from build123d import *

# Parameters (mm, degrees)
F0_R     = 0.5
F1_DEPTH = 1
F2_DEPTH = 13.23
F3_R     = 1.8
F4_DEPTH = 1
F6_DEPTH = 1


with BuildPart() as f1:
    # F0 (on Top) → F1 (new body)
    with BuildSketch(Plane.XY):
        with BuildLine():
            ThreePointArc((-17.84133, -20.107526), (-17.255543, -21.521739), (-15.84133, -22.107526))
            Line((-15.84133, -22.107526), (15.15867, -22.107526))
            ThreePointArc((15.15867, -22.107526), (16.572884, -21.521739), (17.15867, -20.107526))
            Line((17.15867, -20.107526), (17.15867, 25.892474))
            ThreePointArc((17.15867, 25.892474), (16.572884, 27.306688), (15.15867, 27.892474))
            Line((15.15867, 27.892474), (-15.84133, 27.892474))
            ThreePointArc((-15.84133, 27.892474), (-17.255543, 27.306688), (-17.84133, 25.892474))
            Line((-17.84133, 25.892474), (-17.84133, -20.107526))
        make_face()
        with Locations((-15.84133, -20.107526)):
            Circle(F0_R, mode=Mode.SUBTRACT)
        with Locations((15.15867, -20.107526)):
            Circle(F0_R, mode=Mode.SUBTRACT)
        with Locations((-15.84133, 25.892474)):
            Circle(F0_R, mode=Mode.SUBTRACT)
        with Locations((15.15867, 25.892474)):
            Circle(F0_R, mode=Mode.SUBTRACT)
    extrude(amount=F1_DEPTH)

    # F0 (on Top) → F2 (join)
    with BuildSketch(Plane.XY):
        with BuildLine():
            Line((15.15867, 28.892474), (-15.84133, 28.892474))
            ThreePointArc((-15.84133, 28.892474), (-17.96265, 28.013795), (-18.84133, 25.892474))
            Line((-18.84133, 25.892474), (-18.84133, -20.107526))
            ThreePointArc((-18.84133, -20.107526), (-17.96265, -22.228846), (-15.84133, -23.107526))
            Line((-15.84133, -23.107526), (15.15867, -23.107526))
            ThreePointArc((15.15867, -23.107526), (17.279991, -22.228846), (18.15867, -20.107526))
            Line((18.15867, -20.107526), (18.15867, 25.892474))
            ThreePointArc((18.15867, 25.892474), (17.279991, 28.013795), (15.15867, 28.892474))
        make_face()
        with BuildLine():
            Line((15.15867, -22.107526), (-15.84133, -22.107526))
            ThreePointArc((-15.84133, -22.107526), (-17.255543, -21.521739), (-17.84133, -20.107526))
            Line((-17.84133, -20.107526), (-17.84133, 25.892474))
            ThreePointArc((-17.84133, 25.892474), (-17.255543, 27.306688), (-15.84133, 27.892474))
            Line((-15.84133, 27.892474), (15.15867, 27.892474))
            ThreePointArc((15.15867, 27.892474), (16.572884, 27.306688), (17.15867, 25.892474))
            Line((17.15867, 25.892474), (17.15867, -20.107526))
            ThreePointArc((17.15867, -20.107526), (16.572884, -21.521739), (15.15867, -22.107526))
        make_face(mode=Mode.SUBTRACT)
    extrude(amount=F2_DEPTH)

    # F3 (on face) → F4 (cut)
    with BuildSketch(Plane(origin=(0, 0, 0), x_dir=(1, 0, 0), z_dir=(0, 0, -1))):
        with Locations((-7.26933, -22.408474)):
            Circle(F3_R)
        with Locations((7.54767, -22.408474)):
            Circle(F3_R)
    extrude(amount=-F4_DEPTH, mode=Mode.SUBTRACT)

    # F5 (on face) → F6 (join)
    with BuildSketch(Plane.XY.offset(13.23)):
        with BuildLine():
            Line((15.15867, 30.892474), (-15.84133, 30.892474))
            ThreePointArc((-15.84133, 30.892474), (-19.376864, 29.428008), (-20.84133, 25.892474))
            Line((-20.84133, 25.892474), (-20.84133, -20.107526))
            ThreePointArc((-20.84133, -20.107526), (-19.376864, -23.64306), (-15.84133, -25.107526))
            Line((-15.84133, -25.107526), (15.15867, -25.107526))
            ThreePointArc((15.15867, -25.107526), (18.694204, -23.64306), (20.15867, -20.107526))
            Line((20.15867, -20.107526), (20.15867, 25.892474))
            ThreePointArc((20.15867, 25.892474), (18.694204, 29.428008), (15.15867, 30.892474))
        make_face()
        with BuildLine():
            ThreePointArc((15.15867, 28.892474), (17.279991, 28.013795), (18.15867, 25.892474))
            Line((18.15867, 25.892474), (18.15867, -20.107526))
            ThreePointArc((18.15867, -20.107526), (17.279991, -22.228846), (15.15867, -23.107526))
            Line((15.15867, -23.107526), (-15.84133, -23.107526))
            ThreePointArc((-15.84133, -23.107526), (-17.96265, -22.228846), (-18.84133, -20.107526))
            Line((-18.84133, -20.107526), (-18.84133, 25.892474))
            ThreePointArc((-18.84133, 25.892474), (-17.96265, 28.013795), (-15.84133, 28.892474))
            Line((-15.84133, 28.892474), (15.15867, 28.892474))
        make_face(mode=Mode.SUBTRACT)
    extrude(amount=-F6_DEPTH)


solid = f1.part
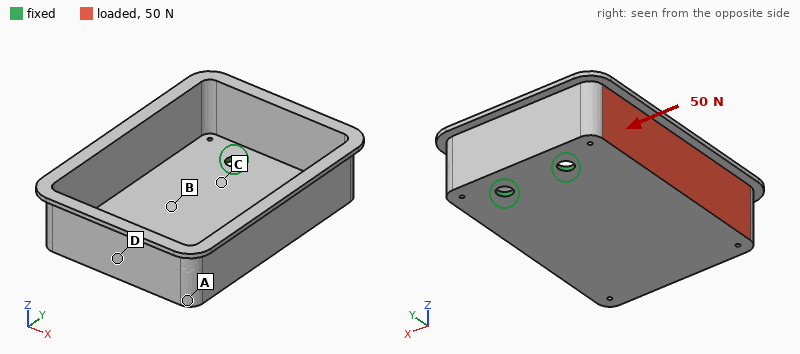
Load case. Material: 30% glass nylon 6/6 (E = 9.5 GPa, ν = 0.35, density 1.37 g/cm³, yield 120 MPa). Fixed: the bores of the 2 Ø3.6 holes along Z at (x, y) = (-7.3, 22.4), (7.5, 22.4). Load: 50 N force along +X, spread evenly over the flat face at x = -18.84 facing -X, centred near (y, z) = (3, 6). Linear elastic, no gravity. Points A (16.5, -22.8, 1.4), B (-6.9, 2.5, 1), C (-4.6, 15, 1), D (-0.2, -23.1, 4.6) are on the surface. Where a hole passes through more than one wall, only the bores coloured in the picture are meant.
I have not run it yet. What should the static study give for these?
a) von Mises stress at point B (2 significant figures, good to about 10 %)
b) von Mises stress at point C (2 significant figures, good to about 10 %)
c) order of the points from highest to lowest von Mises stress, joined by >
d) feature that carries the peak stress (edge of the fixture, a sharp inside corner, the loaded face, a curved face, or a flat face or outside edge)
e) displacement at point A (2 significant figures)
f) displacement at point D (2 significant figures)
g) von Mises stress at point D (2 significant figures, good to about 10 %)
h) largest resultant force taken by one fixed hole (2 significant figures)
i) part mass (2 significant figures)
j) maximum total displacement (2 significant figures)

7.4 MPa
9.8 MPa
C > B > D > A
a curved face
0.32 mm
0.20 mm
3.5 MPa
62 N
5.9 g
0.79 mm
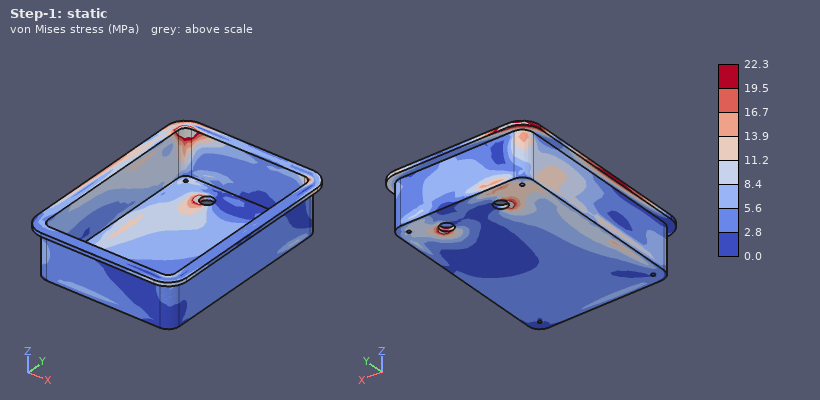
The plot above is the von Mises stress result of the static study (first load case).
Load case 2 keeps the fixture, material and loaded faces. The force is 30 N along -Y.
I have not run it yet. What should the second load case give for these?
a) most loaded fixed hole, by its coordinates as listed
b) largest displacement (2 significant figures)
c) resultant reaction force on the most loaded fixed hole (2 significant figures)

(-7.3, 22.4)
0.83 mm
47 N
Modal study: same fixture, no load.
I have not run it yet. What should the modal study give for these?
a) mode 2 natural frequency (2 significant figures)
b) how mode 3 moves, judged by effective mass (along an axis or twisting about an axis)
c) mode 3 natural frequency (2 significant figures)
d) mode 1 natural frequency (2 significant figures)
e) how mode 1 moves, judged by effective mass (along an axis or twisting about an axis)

520 Hz
along X
2100 Hz
270 Hz
along Z
